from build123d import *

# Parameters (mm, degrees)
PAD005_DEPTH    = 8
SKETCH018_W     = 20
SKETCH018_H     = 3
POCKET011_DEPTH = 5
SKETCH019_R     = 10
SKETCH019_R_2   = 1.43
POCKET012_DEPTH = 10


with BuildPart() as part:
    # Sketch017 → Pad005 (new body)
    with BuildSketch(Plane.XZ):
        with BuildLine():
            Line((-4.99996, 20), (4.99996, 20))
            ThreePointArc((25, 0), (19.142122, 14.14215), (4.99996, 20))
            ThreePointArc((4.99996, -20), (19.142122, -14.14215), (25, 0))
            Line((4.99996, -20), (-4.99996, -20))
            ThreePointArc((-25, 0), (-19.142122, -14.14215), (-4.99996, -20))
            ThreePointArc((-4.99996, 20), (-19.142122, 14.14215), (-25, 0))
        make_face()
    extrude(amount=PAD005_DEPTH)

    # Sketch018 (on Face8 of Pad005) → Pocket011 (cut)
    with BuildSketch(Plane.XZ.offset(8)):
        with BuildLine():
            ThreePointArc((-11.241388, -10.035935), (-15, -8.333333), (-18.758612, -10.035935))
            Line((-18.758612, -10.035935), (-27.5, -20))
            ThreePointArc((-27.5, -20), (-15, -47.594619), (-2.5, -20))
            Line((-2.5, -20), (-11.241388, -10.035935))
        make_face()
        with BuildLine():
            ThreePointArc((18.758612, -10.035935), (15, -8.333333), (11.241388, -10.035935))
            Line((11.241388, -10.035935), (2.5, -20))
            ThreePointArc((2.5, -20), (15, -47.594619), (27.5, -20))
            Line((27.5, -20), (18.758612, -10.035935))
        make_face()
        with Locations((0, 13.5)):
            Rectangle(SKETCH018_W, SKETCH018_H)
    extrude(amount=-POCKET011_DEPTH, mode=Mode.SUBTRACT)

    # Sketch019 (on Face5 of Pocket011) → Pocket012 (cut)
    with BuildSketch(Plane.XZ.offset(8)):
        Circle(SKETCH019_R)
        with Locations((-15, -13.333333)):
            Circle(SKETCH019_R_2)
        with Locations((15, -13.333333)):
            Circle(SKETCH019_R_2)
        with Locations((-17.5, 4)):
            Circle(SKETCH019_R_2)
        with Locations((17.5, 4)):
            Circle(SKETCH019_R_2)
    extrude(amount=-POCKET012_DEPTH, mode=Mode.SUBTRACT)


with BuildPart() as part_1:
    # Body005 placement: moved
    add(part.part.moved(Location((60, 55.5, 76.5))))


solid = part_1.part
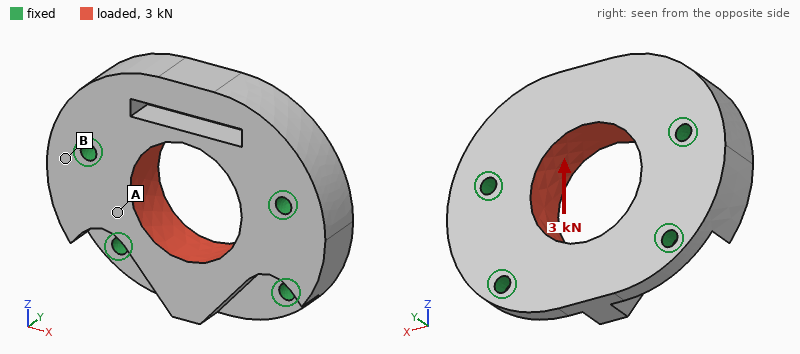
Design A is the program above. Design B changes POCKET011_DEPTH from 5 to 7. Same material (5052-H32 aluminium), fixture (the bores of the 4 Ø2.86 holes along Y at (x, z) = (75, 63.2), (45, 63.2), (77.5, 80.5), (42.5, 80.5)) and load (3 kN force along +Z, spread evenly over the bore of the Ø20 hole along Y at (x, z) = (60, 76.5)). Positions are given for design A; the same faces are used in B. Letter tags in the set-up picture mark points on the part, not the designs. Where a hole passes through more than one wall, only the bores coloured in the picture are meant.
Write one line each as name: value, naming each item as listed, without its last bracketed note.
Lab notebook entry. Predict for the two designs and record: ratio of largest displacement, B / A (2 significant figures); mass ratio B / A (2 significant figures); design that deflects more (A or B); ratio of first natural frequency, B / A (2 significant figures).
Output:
ratio of largest displacement, B / A: 1.3
mass ratio B / A: 0.94
design that deflects more: B
ratio of first natural frequency, B / A: 0.78
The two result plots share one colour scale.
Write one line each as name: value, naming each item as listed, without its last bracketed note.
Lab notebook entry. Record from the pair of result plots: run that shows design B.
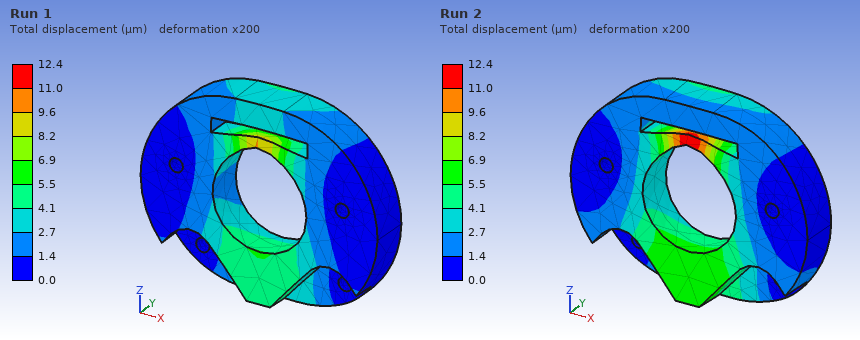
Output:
run that shows design B: Run 2
